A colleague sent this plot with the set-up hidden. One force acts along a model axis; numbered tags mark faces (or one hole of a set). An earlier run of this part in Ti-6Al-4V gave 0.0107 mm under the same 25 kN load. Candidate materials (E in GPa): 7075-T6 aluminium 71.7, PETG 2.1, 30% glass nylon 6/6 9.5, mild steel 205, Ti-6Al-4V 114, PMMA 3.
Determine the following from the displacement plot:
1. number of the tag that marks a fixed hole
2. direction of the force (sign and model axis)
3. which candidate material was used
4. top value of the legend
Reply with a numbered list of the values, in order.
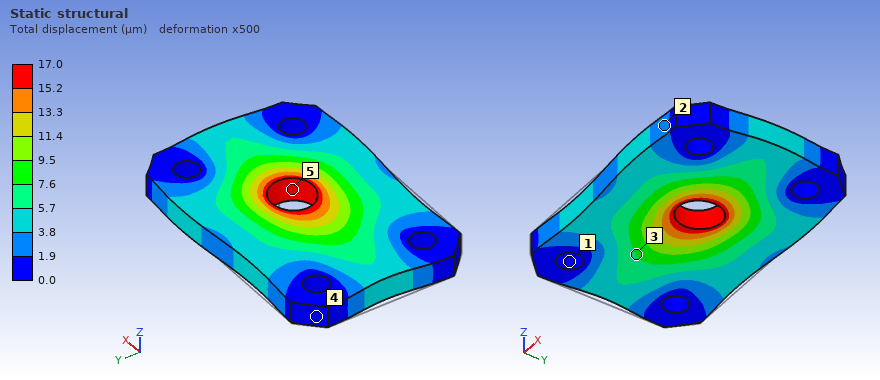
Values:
1. 1
2. +X
3. 7075-T6 aluminium
4. 17.0 µm
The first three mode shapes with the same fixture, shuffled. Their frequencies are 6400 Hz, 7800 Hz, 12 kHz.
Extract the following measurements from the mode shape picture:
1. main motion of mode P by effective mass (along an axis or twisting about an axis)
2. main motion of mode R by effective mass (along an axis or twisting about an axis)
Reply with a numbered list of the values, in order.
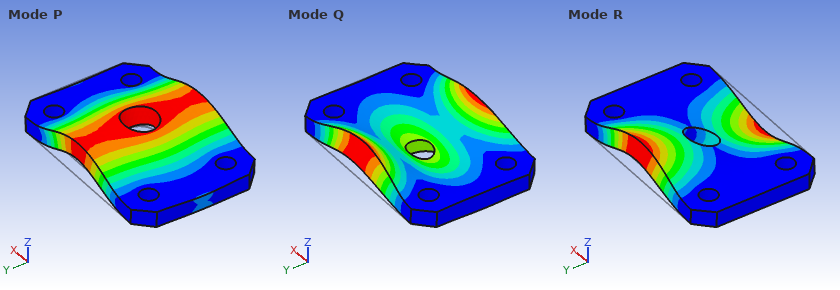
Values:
1. along Z
2. twisting about X
